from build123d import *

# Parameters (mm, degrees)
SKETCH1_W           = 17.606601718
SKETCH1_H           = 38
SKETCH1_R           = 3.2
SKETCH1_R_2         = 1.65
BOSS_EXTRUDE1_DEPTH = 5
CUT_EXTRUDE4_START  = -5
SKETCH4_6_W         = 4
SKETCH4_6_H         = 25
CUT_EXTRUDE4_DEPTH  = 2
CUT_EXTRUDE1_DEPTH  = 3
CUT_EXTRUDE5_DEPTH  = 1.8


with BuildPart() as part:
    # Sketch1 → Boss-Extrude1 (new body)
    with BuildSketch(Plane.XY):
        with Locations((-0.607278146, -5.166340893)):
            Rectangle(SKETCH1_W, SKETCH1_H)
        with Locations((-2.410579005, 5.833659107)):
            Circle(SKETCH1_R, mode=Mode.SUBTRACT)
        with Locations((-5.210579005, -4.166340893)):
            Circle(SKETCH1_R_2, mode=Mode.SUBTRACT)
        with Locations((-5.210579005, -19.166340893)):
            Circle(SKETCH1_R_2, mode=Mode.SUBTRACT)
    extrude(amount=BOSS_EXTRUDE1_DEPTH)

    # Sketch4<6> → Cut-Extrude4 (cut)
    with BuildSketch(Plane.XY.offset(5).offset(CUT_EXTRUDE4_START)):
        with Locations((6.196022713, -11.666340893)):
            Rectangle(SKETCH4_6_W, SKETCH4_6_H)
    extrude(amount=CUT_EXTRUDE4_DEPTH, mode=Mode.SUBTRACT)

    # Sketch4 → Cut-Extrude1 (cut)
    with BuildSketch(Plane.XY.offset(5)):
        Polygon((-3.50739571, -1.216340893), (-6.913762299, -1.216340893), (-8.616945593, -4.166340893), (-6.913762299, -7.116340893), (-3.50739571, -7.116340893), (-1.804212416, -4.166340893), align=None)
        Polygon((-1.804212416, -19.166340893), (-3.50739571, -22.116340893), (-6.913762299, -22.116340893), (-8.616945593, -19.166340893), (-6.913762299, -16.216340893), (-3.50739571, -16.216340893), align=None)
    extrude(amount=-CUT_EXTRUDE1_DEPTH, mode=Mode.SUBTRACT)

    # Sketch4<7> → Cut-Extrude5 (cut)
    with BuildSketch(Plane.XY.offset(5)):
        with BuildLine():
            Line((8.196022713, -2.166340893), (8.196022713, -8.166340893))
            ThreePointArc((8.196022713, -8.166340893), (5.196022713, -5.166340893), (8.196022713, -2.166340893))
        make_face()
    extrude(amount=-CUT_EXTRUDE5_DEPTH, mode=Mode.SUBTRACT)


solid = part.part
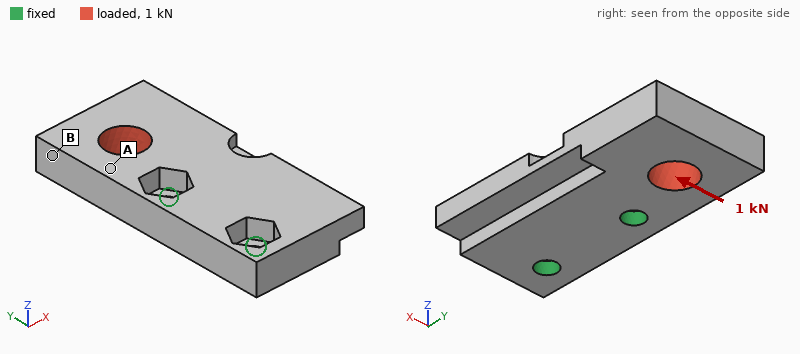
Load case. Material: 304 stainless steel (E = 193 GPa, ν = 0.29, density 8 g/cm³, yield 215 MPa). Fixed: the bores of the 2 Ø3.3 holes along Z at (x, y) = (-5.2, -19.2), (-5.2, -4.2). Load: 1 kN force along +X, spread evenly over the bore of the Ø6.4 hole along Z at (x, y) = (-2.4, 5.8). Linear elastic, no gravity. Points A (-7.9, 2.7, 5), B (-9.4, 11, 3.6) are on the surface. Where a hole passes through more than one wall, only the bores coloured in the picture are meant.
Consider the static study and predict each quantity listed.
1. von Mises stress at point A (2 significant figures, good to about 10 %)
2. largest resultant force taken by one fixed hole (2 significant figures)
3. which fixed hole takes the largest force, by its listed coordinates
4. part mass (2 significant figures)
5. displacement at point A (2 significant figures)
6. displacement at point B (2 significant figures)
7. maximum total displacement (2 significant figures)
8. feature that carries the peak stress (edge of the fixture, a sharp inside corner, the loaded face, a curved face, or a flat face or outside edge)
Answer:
35 MPa
1.5 kN
(-5.2, -4.2)
22 g
8.4 µm
14 µm
23 µm
edge of the fixture
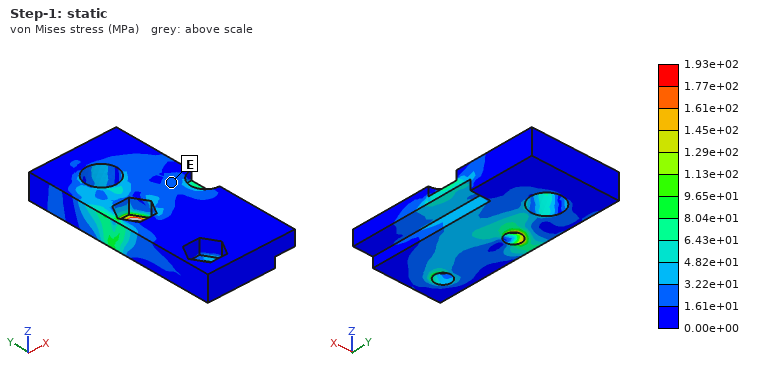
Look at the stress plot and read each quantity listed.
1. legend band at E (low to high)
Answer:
1.61e+01 to 3.22e+01 MPa
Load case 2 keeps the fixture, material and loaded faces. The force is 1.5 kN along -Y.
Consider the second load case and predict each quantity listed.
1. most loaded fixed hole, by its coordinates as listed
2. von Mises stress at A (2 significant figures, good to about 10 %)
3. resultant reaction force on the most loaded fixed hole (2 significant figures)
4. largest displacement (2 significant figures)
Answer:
(-5.2, -4.2)
20 MPa
1.1 kN
8.2 µm
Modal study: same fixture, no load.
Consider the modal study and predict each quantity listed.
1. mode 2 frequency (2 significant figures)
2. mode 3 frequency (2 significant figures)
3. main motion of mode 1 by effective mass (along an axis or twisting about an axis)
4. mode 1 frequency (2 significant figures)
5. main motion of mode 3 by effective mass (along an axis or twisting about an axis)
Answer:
11 kHz
15 kHz
along Z
6600 Hz
along X
